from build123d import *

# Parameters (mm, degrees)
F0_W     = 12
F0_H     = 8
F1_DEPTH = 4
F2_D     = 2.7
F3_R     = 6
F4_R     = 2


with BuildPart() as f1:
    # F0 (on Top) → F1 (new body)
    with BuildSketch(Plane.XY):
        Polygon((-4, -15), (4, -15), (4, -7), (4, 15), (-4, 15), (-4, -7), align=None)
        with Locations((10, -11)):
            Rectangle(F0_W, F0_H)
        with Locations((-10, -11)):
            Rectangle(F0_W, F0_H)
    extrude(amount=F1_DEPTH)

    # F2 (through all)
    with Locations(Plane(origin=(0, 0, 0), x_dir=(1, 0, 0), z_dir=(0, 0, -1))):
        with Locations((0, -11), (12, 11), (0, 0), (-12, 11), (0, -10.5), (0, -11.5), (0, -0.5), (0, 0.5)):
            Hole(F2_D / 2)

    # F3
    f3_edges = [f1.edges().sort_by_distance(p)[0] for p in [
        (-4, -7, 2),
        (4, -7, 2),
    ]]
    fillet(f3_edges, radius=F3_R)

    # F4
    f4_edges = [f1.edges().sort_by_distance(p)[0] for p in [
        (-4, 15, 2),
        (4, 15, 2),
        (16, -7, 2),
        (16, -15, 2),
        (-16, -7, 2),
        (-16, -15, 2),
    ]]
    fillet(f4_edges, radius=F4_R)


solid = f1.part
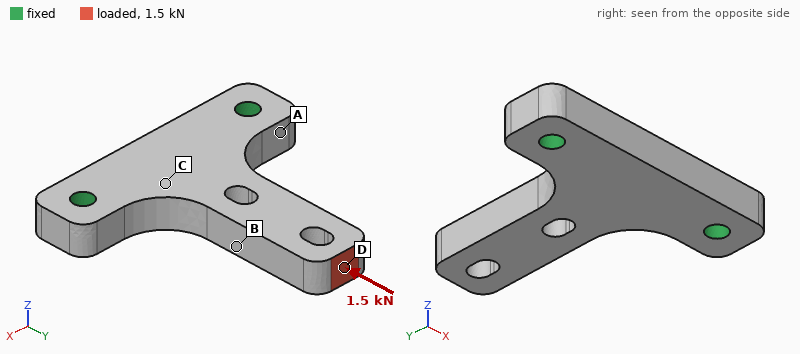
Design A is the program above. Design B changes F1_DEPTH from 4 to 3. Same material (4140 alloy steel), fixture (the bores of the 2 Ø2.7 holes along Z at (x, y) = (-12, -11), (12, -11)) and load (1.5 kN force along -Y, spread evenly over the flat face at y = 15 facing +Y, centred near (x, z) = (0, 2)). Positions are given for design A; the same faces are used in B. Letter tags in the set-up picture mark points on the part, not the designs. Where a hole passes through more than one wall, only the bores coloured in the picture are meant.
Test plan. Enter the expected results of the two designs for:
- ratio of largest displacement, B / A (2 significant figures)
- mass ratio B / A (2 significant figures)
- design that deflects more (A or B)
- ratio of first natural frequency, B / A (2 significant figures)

1.3
0.75
B
0.78
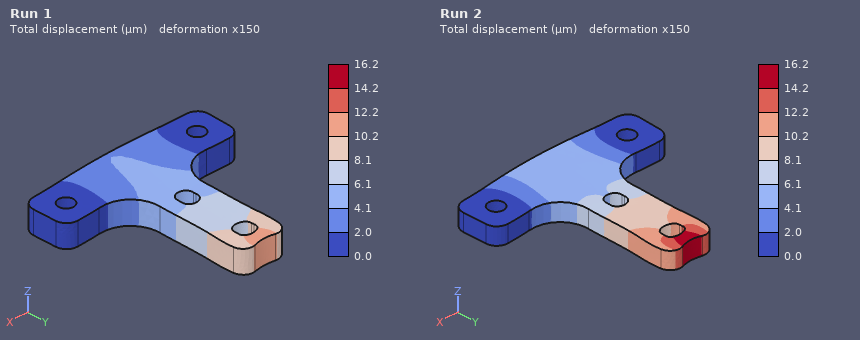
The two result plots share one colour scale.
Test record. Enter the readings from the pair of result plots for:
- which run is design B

Run 2
